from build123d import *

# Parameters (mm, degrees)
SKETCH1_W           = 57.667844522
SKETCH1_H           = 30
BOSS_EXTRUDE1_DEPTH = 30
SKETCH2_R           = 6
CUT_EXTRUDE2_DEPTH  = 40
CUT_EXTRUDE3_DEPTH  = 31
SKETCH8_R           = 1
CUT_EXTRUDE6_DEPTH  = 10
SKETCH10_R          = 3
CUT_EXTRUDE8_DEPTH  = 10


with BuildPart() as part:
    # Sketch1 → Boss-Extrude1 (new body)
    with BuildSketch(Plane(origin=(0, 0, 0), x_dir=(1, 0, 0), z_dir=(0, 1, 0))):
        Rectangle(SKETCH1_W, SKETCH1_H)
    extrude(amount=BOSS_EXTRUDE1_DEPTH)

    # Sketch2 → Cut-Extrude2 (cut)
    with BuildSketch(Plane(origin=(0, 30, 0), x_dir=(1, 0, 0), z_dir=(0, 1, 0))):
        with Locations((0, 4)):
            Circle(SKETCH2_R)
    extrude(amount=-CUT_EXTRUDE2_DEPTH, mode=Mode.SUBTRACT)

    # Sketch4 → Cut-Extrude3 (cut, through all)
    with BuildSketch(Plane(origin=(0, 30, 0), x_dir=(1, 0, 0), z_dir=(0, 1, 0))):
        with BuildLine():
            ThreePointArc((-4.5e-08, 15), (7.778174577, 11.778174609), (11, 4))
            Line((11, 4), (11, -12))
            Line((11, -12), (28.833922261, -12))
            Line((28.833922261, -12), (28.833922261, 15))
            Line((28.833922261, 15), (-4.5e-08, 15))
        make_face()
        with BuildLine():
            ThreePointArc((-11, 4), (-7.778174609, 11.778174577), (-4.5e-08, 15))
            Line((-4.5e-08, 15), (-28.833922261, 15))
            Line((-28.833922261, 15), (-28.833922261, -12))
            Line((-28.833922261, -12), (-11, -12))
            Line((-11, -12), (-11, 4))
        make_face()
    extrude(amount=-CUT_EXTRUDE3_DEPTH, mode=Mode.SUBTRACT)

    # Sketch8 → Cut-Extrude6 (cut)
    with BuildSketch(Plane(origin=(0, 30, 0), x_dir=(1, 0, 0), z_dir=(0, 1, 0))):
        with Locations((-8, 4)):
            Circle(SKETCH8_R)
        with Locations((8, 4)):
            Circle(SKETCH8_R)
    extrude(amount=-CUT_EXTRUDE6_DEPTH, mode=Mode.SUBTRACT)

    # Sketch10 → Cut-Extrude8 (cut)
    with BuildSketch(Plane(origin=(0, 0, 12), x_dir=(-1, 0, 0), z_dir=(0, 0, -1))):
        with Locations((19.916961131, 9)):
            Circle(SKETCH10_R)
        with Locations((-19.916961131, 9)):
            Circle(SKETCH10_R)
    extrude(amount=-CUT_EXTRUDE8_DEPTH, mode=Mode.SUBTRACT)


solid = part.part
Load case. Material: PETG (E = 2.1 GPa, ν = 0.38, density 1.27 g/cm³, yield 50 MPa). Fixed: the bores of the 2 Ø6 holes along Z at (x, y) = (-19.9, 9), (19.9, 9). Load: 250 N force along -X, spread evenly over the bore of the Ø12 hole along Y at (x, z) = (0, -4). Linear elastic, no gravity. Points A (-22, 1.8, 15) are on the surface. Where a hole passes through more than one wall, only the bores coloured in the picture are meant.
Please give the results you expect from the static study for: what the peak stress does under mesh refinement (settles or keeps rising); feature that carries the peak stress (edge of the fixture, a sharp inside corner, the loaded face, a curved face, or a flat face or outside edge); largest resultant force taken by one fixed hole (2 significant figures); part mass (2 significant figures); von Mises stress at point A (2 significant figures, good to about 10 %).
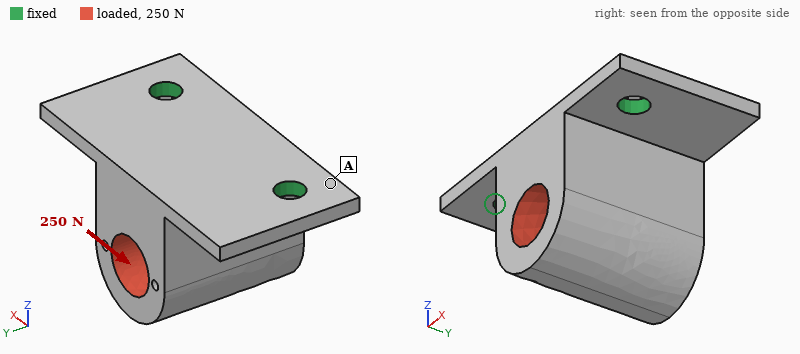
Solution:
keeps rising
edge of the fixture
200 N
23 g
3.2 MPa
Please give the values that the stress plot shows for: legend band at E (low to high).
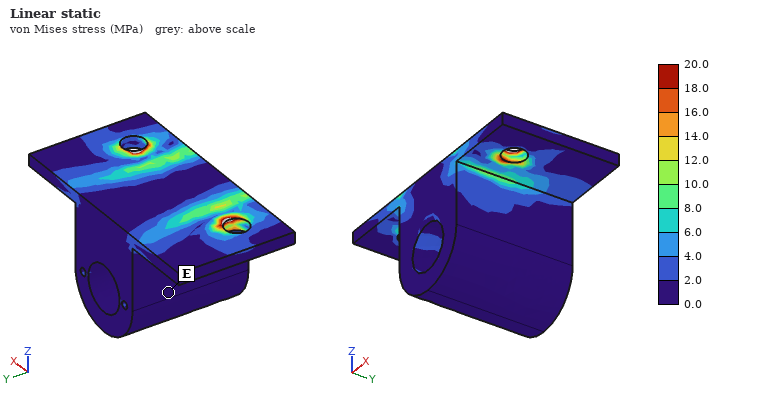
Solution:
0.0 to 2.0 MPa
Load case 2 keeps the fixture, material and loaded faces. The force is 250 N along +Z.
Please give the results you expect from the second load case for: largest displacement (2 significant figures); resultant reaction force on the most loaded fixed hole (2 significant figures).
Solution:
0.75 mm
130 N
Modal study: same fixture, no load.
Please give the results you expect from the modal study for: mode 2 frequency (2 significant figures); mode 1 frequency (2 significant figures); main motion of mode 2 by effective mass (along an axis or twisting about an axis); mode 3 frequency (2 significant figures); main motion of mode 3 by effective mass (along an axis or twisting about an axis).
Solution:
1600 Hz
540 Hz
along X
1800 Hz
along Z
